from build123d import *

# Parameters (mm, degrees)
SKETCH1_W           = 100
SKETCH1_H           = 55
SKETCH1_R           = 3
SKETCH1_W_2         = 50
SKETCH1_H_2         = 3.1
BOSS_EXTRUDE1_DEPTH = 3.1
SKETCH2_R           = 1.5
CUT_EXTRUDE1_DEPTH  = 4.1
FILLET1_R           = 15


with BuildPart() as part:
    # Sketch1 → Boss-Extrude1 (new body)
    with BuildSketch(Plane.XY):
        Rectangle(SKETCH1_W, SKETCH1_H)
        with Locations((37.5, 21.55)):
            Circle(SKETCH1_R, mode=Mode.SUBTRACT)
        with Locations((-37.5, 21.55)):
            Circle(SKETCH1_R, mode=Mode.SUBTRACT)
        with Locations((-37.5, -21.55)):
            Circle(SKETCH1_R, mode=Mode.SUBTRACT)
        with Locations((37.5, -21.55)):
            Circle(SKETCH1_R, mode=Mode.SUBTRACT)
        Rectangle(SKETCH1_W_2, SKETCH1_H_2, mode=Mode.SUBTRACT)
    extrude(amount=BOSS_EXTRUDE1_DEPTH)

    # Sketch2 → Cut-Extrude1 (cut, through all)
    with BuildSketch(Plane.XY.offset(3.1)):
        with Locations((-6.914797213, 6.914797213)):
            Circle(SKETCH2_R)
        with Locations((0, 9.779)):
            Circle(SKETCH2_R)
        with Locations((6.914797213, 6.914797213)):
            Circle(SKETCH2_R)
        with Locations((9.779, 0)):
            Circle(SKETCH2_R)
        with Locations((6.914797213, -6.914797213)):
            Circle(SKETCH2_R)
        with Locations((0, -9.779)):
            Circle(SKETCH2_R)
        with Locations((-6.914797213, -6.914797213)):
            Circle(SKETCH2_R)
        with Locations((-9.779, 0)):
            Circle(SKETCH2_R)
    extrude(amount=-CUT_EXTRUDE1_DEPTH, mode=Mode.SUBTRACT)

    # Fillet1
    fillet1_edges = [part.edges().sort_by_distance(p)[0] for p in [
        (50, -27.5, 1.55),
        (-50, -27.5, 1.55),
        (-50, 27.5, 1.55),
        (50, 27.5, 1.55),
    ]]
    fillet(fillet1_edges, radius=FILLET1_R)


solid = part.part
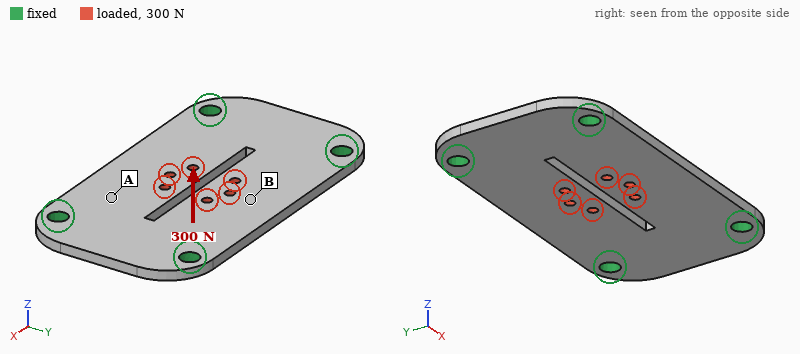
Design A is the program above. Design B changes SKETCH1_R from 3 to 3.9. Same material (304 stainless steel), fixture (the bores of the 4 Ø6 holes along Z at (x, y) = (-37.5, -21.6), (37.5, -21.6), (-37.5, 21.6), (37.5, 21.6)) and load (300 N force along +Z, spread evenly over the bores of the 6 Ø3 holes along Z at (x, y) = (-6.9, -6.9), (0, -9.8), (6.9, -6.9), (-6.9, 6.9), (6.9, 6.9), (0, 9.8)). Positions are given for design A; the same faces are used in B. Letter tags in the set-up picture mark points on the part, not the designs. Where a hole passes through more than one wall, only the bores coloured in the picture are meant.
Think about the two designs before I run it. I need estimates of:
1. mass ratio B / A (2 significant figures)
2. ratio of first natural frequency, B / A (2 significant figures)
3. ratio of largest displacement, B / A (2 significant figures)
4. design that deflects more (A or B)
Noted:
0.98
1.1
0.92
A
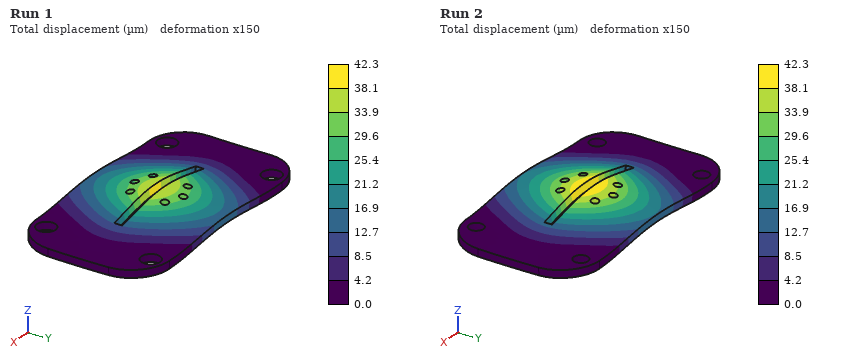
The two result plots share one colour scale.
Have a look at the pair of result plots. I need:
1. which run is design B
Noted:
Run 1
